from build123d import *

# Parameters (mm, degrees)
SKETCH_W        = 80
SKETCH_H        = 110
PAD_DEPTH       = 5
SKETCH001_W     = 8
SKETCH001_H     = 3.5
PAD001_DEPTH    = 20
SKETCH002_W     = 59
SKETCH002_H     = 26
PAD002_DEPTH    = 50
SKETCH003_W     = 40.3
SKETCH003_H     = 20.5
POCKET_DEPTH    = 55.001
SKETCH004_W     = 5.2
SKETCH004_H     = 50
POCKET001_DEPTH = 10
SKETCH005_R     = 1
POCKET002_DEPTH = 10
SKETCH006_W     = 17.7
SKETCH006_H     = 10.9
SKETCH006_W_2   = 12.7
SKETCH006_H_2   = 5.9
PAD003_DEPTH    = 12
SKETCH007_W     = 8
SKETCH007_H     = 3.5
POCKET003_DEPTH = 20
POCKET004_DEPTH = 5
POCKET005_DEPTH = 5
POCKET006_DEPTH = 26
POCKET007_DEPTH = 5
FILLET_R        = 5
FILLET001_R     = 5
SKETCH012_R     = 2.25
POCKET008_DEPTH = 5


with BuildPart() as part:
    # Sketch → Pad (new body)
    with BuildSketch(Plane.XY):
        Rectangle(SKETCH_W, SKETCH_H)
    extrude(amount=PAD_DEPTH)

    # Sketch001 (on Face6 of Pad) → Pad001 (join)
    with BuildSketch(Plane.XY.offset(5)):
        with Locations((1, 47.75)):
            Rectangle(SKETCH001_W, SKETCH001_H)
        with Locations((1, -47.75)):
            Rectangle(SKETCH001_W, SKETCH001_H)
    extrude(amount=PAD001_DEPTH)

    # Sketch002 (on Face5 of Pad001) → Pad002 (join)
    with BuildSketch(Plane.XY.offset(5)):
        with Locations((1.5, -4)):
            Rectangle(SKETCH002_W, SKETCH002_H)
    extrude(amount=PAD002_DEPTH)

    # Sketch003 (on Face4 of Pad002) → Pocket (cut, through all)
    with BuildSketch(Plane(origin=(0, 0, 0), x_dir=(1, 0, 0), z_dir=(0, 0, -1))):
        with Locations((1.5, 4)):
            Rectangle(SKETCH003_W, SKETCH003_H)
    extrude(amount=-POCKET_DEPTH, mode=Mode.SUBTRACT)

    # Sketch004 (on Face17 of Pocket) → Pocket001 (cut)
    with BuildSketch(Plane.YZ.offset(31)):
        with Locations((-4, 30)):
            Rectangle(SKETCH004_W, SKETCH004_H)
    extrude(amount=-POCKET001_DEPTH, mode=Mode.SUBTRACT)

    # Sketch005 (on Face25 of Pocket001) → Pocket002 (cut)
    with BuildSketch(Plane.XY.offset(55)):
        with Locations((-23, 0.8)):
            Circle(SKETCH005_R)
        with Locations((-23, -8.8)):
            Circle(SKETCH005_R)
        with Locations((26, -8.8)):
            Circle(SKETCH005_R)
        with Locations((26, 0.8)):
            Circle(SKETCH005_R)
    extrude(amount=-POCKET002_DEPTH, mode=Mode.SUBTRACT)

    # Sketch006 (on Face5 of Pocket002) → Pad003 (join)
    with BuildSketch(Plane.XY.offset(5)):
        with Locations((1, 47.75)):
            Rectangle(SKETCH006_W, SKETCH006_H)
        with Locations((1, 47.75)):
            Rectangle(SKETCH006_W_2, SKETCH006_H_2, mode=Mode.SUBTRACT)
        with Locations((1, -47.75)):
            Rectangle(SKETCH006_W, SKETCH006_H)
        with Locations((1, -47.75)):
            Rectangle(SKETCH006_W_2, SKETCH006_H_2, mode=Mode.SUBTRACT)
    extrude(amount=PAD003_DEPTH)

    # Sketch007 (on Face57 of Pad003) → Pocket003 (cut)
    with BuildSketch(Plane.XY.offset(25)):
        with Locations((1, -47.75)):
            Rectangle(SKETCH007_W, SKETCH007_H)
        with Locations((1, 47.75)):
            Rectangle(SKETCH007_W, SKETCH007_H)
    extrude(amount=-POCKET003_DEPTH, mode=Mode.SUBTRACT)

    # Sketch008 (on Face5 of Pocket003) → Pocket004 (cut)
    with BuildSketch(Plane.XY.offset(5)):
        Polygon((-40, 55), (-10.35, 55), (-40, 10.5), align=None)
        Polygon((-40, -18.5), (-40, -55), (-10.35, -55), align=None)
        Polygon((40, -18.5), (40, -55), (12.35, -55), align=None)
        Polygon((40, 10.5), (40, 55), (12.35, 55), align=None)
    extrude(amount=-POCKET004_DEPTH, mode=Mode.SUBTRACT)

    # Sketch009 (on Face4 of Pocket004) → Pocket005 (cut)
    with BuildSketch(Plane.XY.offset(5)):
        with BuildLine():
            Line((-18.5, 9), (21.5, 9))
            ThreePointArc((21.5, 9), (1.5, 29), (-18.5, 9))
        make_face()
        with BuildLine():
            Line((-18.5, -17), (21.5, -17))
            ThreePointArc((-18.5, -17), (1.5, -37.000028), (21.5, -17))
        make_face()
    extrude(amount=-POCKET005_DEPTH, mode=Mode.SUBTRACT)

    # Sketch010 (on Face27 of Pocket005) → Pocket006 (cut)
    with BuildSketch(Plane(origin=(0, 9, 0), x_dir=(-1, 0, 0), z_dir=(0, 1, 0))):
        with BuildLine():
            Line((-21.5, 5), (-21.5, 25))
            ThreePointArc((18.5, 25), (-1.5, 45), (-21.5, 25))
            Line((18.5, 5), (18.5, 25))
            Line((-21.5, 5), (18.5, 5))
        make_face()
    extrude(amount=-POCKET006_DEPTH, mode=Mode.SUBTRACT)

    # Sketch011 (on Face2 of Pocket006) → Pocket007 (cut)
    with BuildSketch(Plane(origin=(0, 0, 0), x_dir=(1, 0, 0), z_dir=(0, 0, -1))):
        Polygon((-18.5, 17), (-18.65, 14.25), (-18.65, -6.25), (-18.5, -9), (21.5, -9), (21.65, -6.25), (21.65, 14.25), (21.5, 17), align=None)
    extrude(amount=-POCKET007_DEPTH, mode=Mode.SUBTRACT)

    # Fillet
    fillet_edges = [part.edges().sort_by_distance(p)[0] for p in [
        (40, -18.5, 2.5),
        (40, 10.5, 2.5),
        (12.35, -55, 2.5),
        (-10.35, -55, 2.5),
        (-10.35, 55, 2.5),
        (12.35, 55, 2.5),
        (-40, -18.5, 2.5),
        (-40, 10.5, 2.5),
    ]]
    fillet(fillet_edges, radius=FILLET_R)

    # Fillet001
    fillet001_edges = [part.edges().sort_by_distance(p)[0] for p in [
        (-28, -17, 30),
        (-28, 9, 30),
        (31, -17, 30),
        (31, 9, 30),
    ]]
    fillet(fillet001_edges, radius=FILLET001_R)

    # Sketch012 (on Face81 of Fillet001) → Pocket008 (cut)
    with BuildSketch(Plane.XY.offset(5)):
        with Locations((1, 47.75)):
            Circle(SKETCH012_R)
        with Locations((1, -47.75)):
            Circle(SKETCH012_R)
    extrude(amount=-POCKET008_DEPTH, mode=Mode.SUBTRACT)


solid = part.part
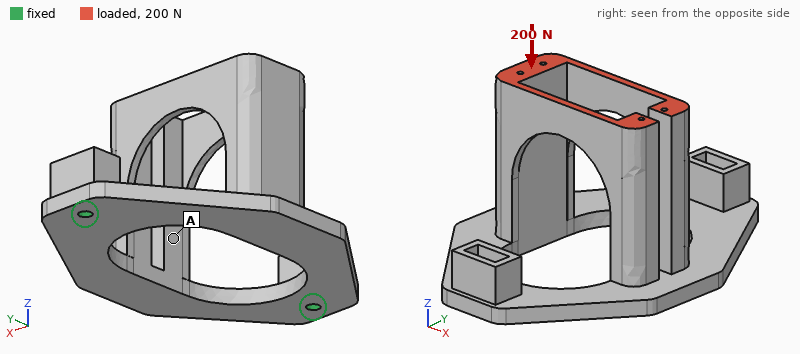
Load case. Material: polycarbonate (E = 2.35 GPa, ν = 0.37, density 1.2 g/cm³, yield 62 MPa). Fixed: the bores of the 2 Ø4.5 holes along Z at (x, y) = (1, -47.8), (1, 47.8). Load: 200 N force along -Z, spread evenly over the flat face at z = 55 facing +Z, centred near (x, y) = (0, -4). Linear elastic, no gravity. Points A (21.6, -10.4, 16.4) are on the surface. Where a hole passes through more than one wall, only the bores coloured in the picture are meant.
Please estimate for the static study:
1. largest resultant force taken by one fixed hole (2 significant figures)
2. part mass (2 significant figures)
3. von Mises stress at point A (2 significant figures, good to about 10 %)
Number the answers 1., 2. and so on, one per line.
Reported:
1. 110 N
2. 57 g
3. 1.9 MPa
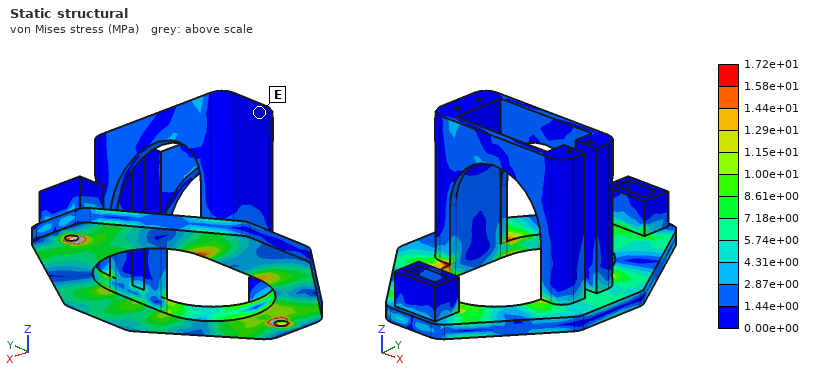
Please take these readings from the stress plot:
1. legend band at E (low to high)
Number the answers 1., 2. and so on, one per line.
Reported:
1. 0.00e+00 to 1.44e+00 MPa
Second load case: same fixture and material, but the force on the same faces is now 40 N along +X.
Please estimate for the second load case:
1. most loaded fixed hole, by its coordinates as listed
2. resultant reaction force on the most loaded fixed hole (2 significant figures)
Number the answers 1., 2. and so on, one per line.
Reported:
1. (1, -47.8)
2. 21 N
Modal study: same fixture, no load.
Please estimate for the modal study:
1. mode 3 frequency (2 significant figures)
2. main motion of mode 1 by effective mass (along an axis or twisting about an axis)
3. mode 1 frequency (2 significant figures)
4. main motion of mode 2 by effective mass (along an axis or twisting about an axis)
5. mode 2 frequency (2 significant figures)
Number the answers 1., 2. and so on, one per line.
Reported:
1. 390 Hz
2. along X
3. 200 Hz
4. along Z
5. 340 Hz
